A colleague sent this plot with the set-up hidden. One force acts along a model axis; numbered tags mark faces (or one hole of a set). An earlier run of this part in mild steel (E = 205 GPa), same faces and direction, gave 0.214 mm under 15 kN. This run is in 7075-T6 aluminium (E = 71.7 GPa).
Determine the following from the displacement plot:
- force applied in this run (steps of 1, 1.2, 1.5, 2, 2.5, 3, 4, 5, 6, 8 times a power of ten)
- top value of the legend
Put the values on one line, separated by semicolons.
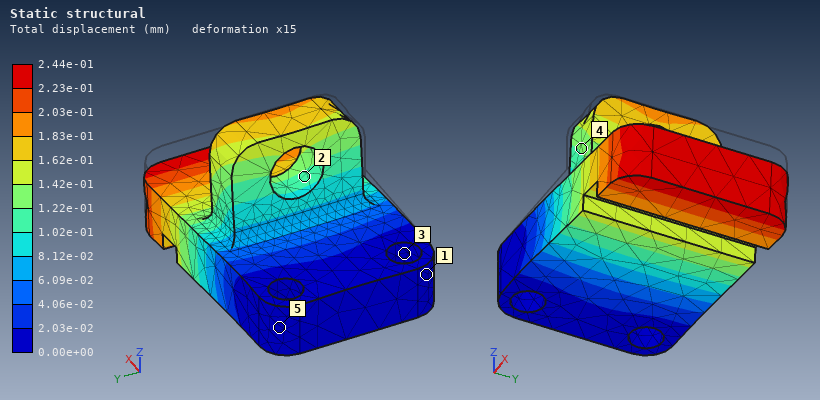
6 kN; 2.44e-01 mm
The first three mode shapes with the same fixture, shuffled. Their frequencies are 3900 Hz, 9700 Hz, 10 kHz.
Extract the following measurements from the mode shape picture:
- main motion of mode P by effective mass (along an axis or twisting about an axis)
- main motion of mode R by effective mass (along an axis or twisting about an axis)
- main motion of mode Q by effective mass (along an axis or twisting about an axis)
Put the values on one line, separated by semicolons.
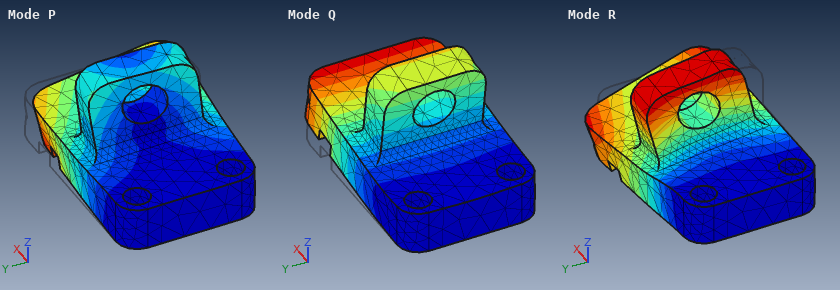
along Y; along Y; along Z
